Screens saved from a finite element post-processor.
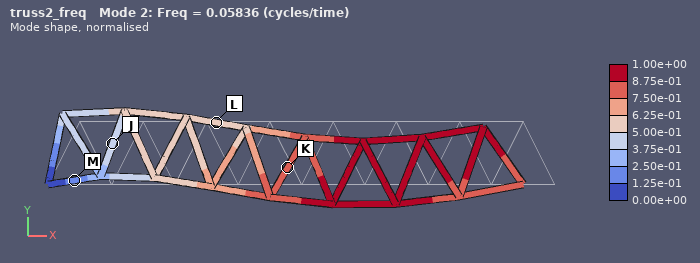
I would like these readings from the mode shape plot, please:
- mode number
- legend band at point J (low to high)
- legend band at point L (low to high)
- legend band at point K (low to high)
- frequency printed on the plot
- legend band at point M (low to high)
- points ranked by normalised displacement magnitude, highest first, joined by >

2
3.75e-01 to 5.00e-01
5.00e-01 to 6.25e-01
7.50e-01 to 8.75e-01
0.05836
1.25e-01 to 2.50e-01
K > L > J > M
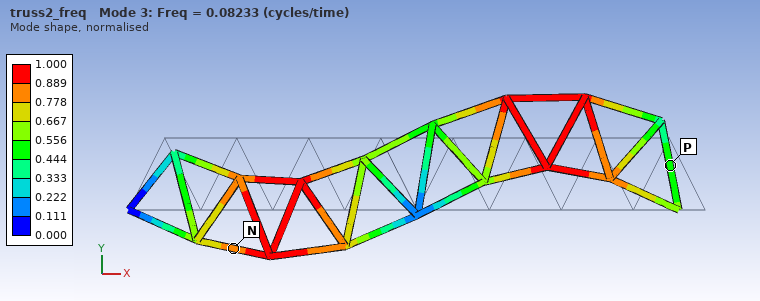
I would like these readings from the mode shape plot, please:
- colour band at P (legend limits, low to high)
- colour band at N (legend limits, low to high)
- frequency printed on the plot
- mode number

0.444 to 0.556
0.778 to 0.889
0.08233
3
